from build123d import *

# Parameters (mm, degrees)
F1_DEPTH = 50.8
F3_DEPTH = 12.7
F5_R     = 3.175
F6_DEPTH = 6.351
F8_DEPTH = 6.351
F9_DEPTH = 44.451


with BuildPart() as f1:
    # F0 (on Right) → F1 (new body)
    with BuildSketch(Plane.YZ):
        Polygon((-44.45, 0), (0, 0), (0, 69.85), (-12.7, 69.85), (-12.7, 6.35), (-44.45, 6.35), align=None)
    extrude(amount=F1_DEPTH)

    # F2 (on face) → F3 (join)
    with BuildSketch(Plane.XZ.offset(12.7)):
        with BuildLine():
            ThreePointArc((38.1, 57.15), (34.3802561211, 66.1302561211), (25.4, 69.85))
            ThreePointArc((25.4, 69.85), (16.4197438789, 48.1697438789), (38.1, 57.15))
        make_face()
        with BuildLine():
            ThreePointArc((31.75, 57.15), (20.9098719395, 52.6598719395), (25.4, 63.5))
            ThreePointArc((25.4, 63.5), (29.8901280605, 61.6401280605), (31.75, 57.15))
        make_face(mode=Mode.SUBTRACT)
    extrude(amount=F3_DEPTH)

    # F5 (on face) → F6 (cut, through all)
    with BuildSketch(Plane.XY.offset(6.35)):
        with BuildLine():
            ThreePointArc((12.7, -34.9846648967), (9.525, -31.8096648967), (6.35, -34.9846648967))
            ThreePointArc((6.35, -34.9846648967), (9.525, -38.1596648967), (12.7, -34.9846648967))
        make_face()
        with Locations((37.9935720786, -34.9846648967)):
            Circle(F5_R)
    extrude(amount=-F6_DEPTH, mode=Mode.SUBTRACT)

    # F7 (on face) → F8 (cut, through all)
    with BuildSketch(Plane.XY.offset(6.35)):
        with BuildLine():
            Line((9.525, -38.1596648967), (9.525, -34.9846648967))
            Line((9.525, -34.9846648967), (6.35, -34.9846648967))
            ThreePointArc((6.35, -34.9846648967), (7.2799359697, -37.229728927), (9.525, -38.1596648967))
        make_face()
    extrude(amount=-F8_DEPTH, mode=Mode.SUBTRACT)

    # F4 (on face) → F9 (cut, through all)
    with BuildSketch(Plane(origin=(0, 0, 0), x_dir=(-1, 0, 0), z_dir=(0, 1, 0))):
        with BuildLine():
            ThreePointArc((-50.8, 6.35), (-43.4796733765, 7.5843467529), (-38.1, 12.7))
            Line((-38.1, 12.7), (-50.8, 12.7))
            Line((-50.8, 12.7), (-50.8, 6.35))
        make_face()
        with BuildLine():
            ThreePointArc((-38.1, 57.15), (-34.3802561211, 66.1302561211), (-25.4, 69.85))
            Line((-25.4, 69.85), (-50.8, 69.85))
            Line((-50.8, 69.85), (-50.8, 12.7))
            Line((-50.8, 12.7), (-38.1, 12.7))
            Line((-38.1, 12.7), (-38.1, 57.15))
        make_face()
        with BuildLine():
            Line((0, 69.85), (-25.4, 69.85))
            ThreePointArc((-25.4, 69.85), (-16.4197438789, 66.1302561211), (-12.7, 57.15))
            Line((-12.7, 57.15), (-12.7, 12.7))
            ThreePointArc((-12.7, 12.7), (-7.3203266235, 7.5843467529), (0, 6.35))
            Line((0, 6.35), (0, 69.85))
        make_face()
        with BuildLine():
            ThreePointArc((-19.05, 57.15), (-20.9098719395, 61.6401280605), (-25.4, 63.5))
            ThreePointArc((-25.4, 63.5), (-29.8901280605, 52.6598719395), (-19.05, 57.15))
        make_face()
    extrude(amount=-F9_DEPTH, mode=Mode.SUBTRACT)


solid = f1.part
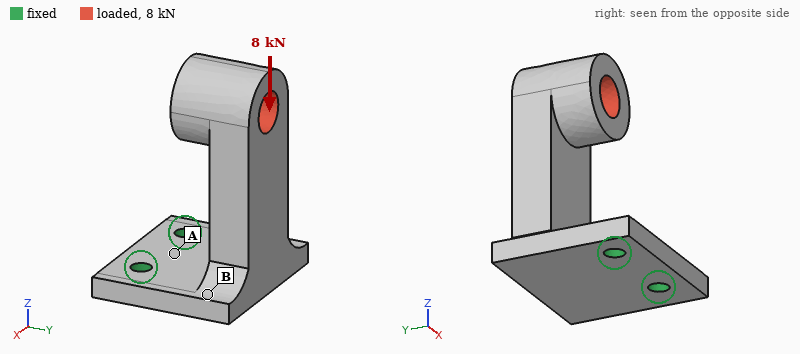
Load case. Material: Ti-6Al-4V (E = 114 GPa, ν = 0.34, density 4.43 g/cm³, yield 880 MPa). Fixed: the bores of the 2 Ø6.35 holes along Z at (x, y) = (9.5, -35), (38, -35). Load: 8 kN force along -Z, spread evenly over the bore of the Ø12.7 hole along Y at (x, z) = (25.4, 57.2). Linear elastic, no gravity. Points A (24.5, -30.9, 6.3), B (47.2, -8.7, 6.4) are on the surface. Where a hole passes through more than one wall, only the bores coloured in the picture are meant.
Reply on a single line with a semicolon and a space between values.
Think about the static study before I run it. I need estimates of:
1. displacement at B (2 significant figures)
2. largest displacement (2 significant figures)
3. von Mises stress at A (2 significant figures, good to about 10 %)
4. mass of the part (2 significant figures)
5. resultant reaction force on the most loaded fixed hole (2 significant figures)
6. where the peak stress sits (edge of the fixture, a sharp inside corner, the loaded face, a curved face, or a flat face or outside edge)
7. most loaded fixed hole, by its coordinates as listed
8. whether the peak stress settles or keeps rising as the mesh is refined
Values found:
0.29 mm; 0.88 mm; 230 MPa; 160 g; 4.4 kN; edge of the fixture; (38, -35); keeps rising
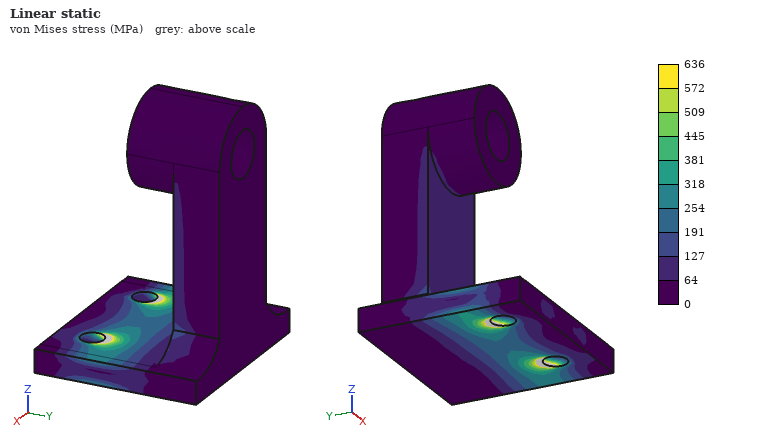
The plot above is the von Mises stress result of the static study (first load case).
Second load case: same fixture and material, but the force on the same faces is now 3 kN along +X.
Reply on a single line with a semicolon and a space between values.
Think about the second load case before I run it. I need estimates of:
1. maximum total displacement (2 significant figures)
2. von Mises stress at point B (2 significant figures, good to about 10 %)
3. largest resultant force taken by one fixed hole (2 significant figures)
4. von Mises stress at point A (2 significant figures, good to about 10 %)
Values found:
0.78 mm; 110 MPa; 5.4 kN; 120 MPa
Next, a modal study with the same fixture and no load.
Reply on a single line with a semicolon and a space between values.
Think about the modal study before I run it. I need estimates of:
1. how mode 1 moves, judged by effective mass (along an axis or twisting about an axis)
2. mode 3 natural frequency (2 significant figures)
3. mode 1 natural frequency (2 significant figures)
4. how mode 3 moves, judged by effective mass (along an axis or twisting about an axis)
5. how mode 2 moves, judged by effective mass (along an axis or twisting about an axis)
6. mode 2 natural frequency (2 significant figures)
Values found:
along Y; 3200 Hz; 770 Hz; along Z; along X; 1500 Hz
